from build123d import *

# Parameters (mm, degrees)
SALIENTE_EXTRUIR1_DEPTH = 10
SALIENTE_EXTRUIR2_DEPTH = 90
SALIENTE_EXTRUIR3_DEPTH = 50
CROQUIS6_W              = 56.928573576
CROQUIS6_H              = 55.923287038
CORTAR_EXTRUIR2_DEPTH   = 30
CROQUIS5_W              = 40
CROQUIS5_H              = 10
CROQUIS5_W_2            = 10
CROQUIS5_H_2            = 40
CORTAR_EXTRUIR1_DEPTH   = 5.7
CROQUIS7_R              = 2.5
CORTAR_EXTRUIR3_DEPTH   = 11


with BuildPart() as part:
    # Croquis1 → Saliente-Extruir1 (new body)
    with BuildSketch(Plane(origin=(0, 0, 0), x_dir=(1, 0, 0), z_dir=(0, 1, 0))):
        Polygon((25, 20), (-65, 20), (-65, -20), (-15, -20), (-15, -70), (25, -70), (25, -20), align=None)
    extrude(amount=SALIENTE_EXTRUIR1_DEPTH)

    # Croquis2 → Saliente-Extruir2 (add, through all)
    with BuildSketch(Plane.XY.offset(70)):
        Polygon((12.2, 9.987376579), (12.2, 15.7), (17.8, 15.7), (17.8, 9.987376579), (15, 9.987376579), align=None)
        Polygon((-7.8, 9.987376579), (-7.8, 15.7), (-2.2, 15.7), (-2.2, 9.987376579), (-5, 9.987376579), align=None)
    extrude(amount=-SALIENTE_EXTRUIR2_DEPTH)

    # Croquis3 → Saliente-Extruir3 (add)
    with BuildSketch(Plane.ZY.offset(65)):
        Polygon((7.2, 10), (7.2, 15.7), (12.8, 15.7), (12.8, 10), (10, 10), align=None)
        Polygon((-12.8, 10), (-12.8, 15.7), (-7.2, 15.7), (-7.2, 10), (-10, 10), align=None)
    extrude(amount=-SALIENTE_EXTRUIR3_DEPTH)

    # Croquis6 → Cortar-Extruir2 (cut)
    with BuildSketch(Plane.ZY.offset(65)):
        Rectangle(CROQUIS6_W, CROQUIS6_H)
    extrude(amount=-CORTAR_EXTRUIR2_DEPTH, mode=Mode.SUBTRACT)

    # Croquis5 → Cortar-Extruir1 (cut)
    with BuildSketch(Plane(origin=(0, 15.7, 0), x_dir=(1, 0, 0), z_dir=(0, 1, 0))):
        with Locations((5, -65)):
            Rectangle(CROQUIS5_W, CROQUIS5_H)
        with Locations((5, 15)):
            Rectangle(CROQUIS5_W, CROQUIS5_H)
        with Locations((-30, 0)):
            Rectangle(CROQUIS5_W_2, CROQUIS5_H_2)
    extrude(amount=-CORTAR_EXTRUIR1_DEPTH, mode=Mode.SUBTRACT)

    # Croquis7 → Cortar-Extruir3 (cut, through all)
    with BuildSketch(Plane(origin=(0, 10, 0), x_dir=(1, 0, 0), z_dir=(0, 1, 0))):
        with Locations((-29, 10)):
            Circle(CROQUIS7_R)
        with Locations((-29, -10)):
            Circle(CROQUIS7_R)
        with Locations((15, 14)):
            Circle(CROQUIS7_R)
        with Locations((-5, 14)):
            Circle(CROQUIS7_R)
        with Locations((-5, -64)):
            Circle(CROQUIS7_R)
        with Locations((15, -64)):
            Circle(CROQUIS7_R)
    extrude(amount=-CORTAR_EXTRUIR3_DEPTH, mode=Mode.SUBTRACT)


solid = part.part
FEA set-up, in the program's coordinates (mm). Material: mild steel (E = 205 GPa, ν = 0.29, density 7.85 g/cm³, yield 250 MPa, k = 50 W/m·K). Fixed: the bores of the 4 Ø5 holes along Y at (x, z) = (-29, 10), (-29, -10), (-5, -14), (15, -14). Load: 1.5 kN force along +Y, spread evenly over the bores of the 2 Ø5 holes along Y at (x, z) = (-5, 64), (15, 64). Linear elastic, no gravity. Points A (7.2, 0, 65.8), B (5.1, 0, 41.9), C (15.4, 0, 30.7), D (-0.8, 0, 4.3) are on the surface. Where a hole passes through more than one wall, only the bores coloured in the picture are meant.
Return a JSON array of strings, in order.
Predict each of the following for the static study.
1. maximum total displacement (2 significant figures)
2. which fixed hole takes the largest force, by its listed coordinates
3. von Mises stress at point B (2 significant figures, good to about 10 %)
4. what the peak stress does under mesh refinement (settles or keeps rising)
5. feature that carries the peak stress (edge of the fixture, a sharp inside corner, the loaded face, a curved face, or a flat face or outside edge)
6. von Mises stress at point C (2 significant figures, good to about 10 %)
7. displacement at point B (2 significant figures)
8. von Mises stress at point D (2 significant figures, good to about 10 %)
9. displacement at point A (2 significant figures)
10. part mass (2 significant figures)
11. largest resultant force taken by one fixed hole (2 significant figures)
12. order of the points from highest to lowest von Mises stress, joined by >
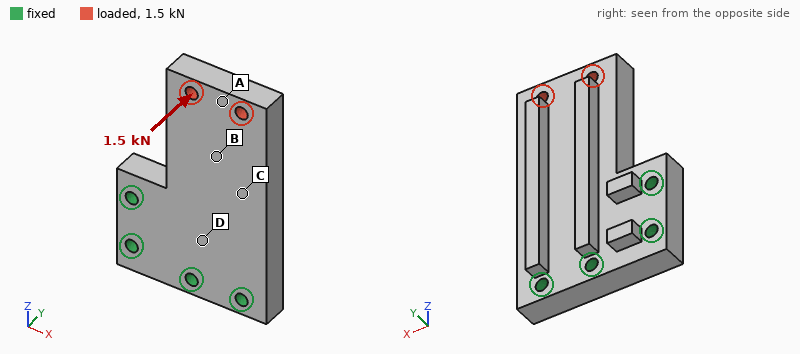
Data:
["0.18 mm", "(-29, 10)", "31 MPa", "keeps rising", "edge of the fixture", "42 MPa", "0.085 mm", "63 MPa", "0.15 mm", "380 g", "2.2 kN", "D > C > B > A"]
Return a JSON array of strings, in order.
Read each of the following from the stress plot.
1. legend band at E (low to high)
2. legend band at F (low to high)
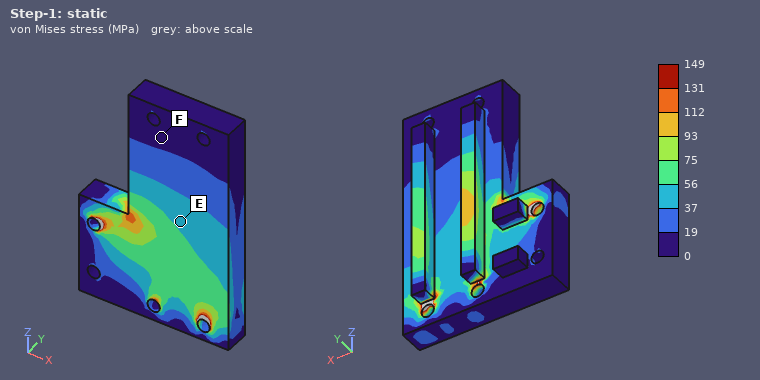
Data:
["37 to 56 MPa", "0 to 19 MPa"]
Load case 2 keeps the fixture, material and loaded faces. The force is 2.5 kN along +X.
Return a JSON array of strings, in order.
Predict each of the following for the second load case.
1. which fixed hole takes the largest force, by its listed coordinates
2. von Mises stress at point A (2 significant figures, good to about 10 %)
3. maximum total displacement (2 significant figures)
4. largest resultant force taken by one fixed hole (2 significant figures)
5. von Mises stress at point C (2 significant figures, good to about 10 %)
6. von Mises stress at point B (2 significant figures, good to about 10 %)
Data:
["(15, -14)", "7.5 MPa", "27 µm", "3.5 kN", "18 MPa", "16 MPa"]
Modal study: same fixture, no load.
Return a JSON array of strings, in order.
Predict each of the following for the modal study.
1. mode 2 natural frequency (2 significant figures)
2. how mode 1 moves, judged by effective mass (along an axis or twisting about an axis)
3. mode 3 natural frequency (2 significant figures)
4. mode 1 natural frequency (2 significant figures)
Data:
["5700 Hz", "along Y", "5900 Hz", "1800 Hz"]
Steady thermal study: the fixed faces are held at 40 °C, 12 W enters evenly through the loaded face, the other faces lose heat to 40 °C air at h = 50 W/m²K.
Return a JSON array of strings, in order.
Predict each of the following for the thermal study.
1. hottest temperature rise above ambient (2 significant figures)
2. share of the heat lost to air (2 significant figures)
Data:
["26 K", "48 %"]
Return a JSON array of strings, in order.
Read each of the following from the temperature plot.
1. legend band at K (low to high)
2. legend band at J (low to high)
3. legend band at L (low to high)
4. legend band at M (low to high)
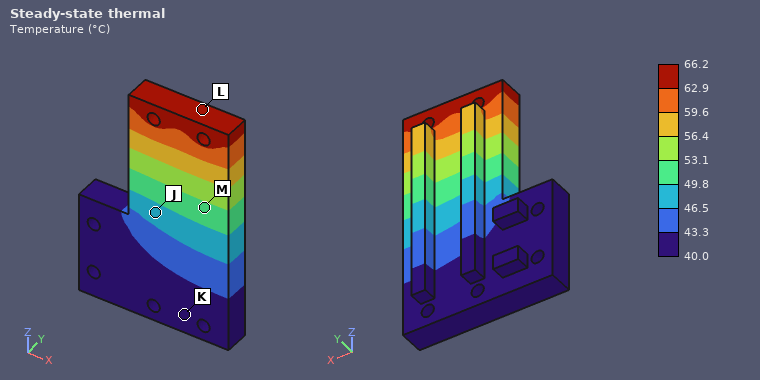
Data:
["40.0 to 43.3 °C", "46.5 to 49.8 °C", "62.9 to 66.2 °C", "49.8 to 53.1 °C"]
